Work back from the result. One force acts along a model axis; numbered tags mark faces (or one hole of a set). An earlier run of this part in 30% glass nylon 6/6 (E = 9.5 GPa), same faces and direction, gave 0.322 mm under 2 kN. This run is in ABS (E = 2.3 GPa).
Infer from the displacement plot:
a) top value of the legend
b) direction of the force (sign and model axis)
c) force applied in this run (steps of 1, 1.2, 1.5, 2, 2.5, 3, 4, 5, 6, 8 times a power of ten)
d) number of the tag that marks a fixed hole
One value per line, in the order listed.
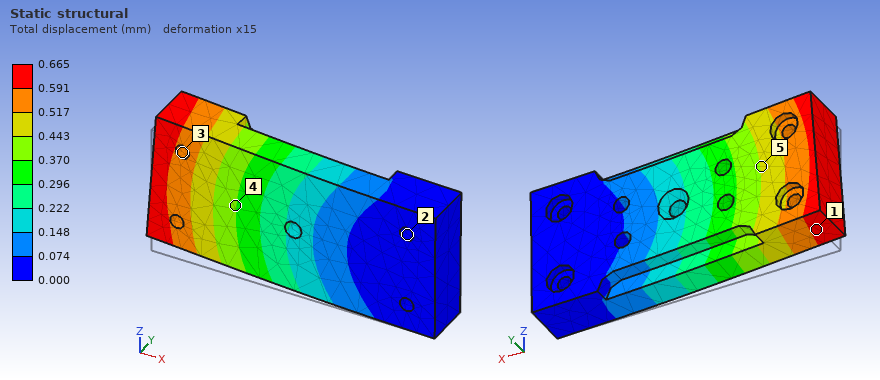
0.665 mm
+Z
1 kN
2
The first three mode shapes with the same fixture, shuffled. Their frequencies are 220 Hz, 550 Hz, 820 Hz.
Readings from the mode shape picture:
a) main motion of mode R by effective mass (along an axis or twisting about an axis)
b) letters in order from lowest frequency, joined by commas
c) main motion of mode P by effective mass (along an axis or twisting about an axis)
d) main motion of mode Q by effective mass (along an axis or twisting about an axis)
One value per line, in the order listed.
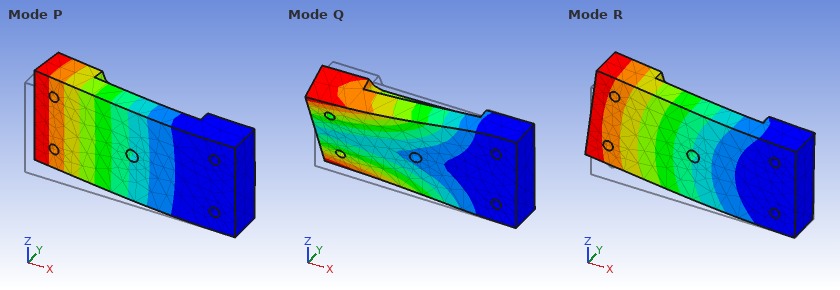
along Z
P, R, Q
along Y
twisting about X
